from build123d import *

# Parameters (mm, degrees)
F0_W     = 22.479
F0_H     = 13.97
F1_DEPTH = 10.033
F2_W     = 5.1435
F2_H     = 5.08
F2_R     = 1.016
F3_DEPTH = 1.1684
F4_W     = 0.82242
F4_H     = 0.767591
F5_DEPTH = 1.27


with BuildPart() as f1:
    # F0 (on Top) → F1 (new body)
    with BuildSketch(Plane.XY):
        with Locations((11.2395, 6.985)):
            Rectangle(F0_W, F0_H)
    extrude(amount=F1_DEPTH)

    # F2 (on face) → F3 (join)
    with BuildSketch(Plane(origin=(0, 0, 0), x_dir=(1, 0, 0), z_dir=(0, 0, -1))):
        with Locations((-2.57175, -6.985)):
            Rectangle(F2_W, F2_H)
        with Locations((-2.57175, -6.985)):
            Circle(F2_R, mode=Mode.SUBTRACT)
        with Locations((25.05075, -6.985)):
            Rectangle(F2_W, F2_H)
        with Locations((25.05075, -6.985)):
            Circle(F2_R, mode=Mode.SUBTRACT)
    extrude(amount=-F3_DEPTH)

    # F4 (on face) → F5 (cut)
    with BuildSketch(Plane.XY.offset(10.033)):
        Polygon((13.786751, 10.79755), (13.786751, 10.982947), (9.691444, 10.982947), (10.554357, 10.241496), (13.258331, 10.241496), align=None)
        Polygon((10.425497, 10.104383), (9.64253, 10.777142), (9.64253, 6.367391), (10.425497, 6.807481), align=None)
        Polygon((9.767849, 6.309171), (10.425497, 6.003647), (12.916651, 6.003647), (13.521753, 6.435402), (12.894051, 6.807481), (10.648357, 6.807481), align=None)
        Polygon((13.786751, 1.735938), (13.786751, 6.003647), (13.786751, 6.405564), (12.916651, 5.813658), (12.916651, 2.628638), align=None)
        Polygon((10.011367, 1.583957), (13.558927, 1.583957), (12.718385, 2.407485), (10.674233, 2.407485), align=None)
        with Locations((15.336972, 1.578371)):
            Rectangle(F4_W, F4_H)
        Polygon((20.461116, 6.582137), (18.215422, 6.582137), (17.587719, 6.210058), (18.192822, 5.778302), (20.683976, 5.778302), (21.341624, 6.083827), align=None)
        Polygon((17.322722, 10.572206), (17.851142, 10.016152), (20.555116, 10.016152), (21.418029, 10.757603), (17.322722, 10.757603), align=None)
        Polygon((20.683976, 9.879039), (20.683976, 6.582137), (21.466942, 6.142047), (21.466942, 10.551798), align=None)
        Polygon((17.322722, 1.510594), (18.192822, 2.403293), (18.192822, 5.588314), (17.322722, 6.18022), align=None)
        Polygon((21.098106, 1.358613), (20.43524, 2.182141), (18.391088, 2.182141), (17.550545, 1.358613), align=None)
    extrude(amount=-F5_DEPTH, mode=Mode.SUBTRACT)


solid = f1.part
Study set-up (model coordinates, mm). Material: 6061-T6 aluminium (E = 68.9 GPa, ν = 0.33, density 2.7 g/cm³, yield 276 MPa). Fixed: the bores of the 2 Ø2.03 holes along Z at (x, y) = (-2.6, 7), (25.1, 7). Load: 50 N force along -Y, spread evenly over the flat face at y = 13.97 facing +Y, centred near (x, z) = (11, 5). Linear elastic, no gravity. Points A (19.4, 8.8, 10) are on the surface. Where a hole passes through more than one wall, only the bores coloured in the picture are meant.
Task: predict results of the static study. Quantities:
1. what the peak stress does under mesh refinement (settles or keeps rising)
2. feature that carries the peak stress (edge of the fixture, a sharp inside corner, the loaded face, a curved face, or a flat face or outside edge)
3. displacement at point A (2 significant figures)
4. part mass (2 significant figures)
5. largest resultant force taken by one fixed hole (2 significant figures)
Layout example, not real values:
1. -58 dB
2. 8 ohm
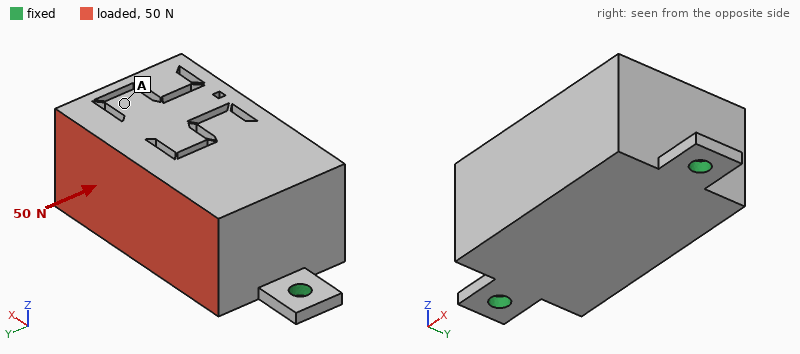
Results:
1. keeps rising
2. edge of the fixture
3. 25 µm
4. 8.6 g
5. 25 N
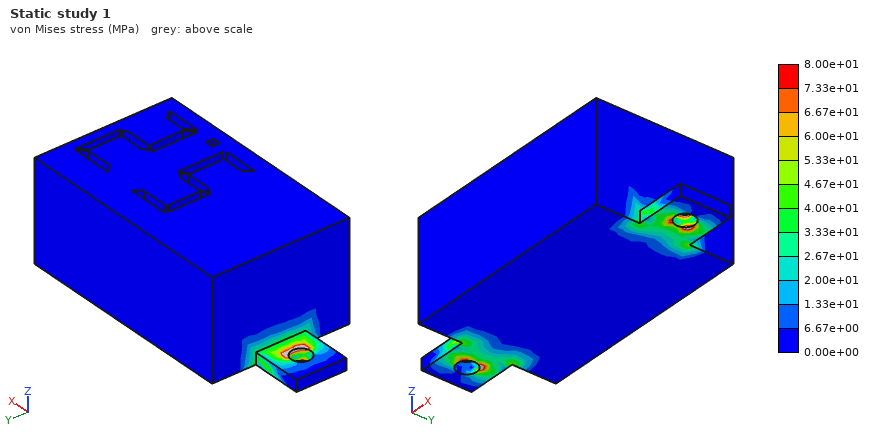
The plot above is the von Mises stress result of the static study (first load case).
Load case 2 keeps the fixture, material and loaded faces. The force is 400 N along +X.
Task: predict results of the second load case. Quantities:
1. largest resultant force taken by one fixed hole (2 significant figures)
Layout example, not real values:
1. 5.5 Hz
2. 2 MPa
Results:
1. 240 N
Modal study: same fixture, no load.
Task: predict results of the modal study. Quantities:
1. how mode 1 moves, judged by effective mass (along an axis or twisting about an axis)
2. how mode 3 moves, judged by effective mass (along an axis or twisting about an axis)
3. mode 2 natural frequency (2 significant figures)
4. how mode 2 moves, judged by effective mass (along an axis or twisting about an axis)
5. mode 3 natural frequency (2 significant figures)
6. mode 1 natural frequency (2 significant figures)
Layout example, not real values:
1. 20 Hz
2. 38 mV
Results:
1. along Y
2. along X
3. 11 kHz
4. along Z
5. 16 kHz
6. 2500 Hz
